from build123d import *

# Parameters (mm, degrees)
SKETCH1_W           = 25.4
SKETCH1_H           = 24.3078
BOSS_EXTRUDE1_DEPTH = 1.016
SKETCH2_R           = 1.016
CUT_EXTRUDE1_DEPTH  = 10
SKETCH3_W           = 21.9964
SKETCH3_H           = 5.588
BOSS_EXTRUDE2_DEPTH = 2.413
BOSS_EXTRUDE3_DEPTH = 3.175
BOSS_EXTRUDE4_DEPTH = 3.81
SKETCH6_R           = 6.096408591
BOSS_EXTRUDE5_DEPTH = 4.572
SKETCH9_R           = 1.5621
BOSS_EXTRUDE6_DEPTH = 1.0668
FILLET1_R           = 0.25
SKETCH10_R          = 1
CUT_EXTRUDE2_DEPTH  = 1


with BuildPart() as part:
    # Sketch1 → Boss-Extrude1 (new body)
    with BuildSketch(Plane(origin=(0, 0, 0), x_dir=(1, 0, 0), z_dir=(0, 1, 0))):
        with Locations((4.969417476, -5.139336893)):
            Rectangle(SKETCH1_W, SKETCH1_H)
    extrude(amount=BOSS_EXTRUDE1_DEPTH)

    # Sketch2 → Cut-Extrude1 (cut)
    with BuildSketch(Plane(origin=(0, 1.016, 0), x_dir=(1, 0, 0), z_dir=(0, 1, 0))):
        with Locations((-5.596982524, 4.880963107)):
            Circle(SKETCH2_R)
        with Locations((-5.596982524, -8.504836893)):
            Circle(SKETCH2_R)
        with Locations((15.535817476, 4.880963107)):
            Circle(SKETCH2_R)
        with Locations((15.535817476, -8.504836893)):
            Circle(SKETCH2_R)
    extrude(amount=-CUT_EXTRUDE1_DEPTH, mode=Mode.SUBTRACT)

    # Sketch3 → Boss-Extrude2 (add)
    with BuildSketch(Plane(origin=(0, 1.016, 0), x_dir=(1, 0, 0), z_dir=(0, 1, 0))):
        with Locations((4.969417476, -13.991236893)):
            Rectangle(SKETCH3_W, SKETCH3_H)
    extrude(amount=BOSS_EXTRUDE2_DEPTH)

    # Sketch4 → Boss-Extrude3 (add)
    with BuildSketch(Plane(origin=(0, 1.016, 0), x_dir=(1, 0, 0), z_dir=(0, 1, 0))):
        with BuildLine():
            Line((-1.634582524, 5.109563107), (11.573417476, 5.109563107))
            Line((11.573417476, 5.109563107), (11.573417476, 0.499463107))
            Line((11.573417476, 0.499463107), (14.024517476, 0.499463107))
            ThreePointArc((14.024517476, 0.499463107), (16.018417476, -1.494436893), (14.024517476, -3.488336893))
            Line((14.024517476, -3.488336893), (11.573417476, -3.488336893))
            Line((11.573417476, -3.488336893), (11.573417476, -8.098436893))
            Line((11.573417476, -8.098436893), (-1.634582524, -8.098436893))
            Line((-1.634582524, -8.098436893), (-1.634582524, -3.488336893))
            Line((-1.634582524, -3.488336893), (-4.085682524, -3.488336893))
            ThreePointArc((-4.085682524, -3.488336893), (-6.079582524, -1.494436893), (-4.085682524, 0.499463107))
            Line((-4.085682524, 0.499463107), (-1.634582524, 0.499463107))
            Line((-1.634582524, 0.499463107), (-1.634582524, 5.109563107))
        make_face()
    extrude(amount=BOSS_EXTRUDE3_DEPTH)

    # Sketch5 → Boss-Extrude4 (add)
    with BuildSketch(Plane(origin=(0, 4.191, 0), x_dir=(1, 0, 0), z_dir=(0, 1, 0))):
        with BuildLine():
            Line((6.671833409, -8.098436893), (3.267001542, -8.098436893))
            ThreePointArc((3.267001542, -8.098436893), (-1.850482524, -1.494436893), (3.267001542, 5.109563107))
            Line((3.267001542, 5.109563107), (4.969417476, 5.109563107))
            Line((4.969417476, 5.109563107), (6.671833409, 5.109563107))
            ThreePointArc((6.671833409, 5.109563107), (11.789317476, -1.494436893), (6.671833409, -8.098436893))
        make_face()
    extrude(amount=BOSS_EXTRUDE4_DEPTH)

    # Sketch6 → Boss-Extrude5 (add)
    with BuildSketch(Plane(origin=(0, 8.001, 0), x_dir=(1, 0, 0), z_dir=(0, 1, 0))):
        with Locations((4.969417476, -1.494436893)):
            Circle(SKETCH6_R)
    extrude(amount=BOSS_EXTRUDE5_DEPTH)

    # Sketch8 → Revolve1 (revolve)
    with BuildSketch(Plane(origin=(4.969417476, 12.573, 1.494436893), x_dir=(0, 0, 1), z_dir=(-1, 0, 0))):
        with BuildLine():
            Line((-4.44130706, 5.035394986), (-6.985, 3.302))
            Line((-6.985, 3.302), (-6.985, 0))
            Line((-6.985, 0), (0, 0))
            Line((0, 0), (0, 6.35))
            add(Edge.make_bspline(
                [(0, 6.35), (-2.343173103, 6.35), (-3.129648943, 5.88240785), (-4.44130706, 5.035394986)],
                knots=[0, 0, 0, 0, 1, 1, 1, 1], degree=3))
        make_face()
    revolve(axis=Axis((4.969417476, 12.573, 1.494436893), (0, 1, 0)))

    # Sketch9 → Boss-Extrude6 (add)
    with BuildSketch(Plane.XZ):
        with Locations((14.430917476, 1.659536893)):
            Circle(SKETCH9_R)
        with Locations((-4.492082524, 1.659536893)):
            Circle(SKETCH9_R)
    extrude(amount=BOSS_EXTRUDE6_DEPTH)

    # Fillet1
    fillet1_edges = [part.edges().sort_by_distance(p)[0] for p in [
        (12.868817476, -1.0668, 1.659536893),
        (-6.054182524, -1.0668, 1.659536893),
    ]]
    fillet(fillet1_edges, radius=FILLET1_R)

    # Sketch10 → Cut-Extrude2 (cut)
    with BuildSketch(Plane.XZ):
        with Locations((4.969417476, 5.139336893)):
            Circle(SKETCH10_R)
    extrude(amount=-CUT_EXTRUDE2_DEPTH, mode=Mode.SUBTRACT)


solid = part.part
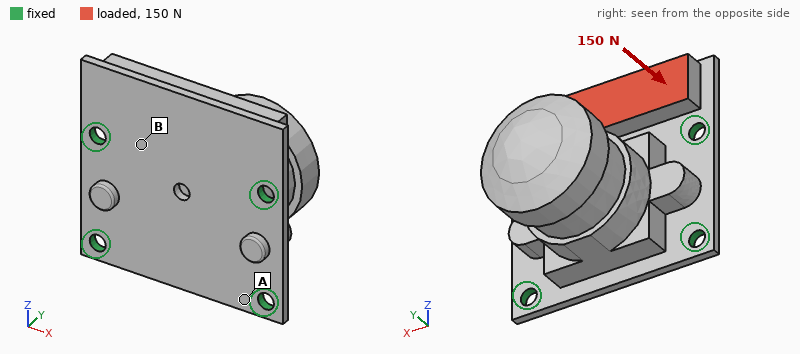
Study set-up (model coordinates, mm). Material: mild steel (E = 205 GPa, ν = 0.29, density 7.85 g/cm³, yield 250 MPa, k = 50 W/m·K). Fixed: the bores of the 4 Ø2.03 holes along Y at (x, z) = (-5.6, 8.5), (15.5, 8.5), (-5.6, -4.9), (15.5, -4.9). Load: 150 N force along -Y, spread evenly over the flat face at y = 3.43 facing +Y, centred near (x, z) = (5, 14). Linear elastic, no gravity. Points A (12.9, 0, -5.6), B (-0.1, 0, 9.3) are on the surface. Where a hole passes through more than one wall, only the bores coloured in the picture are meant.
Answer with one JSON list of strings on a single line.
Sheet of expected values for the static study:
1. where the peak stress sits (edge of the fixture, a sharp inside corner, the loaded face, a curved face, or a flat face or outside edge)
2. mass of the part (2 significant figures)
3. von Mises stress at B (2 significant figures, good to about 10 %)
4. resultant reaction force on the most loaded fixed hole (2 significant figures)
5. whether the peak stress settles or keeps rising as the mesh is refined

["edge of the fixture", "27 g", "87 MPa", "100 N", "keeps rising"]
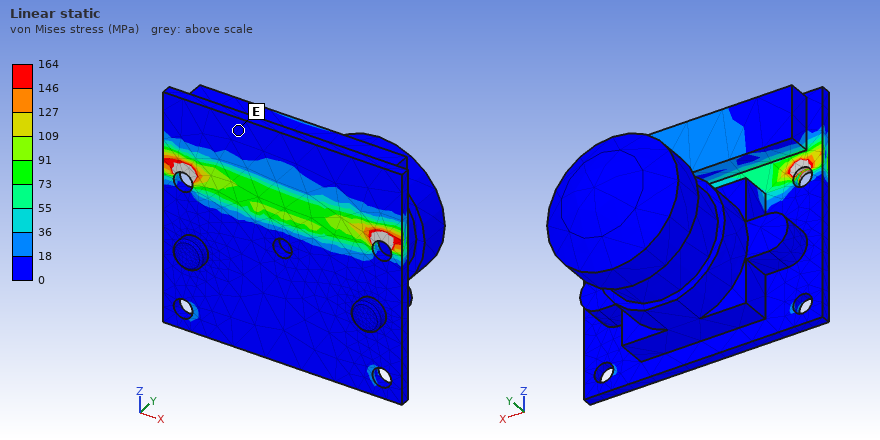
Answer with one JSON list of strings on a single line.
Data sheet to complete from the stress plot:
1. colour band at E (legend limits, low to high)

["0 to 18 MPa"]
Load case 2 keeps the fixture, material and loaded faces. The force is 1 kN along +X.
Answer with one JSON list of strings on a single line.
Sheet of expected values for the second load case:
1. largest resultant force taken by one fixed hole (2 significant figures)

["520 N"]
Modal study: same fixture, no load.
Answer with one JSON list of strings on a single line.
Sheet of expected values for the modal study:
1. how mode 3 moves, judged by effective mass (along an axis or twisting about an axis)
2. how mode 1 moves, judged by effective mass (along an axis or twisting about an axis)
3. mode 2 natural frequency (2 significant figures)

["along X", "along Z", "7100 Hz"]
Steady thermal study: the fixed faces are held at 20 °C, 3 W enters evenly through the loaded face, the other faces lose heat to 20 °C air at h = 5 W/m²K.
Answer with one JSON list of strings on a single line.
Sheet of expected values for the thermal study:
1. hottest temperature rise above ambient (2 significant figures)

["15 K"]
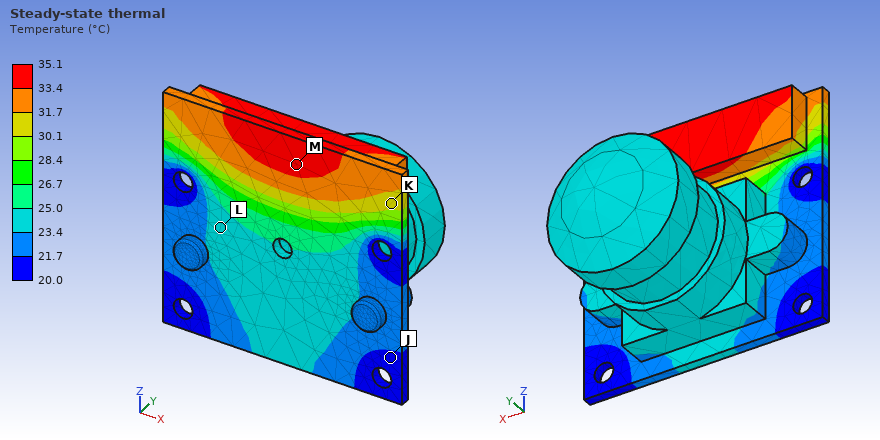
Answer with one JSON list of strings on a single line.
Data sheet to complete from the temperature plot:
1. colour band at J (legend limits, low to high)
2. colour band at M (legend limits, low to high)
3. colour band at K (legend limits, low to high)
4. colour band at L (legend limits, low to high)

["20.0 to 21.7 °C", "33.4 to 35.1 °C", "30.1 to 31.7 °C", "23.4 to 25.0 °C"]
